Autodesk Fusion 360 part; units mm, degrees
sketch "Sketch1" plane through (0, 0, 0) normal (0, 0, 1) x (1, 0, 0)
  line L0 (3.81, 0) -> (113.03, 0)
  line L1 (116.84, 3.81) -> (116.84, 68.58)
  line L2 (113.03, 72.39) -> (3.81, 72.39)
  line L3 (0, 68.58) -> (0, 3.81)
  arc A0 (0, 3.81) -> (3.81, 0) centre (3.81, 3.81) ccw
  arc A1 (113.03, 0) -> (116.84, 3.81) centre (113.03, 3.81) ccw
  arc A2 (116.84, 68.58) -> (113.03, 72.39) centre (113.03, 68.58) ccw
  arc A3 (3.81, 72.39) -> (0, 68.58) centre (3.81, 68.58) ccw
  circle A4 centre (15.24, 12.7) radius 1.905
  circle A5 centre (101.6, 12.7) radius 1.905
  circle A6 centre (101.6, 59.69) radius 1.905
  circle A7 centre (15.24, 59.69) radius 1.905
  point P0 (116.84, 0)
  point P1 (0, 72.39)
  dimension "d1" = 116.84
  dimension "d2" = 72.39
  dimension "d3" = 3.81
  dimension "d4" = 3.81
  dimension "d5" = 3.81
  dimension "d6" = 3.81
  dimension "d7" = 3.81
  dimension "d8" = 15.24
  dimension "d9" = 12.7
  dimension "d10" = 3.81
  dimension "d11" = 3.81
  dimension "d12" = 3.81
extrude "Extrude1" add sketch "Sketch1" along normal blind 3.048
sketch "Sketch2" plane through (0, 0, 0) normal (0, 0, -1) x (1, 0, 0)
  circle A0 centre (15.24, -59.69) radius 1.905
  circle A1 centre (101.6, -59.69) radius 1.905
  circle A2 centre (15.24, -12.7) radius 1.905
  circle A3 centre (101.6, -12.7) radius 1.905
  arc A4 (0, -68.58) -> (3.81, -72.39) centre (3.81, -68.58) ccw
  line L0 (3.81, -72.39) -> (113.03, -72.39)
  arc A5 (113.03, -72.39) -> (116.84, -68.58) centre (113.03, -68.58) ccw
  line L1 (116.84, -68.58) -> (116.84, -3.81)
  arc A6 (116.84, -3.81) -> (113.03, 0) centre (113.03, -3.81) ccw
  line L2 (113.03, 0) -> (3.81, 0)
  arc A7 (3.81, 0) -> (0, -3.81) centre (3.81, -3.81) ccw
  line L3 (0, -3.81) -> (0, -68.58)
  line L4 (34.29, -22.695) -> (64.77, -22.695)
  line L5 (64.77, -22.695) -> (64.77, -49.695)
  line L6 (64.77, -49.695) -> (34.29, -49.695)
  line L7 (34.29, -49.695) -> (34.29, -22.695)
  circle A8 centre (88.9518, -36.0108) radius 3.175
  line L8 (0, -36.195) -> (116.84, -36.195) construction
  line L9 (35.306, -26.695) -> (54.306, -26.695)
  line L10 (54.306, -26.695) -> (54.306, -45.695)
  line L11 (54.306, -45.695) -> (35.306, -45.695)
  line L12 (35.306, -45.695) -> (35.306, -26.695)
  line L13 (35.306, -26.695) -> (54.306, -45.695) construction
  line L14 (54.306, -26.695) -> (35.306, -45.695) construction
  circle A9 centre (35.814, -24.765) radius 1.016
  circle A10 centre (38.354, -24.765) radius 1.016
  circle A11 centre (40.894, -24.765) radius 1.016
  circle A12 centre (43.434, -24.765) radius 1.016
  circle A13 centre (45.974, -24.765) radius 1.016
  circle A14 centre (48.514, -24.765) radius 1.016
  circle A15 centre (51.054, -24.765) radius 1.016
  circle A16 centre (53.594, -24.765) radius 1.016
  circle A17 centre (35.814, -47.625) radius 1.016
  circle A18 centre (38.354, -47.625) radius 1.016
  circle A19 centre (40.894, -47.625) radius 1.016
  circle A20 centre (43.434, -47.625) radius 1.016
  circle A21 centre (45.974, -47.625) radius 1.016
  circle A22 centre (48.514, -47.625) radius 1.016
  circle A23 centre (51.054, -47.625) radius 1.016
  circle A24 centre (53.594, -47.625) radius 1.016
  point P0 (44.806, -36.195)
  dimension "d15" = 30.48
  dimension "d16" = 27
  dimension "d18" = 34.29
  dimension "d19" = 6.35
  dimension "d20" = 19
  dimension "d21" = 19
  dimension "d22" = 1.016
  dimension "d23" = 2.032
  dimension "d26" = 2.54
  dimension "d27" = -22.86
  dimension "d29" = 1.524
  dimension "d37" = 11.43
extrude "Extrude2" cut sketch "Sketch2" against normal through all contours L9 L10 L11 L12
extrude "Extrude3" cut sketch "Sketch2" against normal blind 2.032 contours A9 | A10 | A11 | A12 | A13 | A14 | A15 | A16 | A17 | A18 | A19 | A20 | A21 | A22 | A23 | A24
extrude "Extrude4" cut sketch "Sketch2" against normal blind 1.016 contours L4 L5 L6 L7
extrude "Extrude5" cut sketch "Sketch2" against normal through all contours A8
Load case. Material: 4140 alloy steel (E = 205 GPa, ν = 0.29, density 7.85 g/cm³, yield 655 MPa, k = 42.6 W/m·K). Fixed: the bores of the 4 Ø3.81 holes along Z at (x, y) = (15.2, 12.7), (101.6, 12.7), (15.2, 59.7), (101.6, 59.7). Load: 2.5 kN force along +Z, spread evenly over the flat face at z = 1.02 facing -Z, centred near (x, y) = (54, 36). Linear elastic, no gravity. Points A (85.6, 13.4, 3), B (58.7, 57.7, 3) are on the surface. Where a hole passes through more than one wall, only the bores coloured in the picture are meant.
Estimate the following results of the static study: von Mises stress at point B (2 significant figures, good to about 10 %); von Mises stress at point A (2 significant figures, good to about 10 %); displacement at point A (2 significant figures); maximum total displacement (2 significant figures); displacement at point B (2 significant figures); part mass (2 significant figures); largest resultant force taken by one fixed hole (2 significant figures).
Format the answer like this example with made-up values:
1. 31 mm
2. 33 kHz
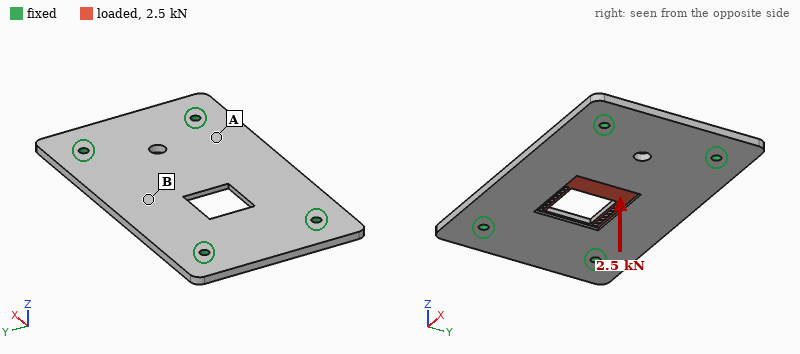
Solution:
1. 220 MPa
2. 86 MPa
3. 0.095 mm
4. 0.53 mm
5. 0.30 mm
6. 190 g
7. 810 N
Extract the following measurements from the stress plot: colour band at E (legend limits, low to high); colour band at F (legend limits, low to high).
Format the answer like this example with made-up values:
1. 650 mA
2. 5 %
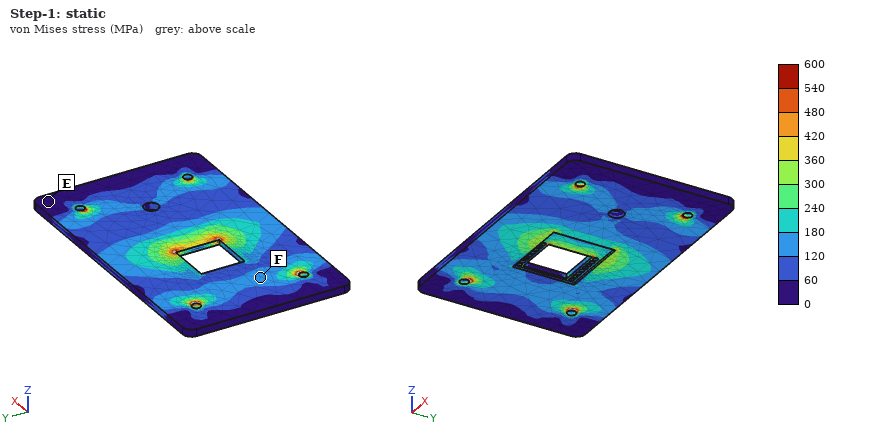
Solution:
1. 0 to 60 MPa
2. 120 to 180 MPa
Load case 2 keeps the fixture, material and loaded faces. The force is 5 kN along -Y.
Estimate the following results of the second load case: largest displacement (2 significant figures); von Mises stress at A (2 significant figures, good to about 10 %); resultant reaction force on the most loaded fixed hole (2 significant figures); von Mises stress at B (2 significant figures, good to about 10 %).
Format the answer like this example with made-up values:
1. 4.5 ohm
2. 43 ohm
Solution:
1. 18 µm
2. 24 MPa
3. 1.9 kN
4. 30 MPa
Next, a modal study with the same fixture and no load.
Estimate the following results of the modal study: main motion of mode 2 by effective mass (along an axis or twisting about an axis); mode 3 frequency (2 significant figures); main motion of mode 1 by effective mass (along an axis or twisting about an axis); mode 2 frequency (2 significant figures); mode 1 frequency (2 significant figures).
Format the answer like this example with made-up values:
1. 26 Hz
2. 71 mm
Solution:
1. twisting about X
2. 4200 Hz
3. along Z
4. 2500 Hz
5. 2000 Hz
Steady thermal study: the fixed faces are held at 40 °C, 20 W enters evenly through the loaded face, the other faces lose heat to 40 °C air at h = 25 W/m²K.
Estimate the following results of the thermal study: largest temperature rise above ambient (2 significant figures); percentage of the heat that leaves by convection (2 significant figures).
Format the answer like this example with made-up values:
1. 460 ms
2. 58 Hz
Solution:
1. 69 K
2. 36 %
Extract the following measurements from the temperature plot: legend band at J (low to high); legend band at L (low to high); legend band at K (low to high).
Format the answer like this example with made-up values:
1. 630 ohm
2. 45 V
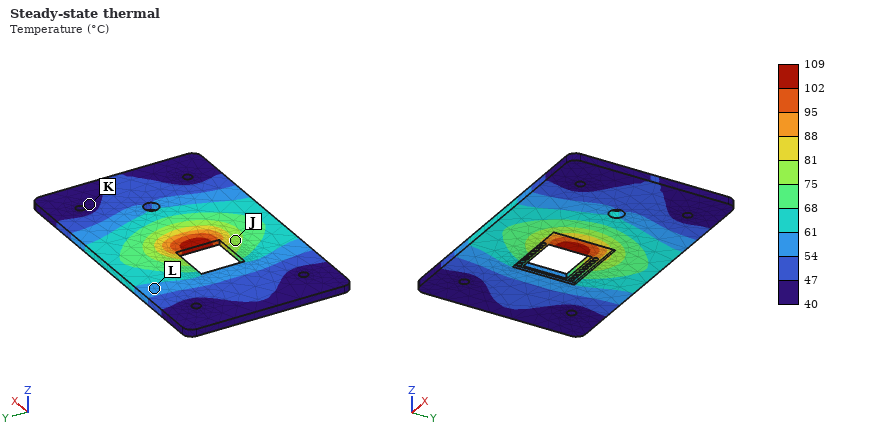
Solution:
1. 75 to 81 °C
2. 54 to 61 °C
3. 40 to 47 °C
